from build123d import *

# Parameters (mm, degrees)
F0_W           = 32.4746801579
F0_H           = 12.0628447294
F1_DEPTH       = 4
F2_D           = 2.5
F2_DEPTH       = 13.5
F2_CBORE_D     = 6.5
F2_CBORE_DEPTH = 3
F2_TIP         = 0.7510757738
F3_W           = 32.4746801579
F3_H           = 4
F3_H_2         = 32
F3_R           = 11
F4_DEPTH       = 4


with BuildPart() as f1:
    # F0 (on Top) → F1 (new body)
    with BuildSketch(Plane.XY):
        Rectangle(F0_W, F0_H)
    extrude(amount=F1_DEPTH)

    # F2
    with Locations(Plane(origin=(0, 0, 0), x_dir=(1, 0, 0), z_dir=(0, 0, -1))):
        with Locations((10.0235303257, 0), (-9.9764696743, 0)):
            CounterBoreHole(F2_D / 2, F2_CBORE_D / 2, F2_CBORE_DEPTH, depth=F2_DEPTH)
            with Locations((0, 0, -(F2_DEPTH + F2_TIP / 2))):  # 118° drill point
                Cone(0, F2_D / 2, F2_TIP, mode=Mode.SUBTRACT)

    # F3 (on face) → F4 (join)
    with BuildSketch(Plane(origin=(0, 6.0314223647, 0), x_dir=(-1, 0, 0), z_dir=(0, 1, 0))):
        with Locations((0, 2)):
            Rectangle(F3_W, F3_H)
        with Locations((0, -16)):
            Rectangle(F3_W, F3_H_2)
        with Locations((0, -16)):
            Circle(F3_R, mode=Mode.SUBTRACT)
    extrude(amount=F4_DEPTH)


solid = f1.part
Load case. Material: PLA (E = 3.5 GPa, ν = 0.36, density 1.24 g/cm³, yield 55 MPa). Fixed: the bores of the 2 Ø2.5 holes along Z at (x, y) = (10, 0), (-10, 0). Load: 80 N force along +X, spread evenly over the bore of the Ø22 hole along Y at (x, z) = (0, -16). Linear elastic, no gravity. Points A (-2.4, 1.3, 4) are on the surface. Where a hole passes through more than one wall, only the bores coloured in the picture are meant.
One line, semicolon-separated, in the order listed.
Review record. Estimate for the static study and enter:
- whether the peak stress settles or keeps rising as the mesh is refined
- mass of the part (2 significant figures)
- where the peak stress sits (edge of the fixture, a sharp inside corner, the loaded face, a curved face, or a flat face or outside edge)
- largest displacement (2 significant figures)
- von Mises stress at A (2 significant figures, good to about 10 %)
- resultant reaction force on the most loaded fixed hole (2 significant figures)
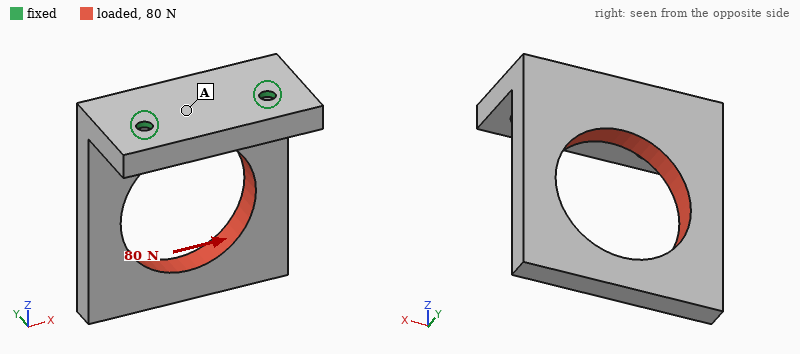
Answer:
keeps rising; 5.6 g; edge of the fixture; 0.46 mm; 4.7 MPa; 91 N
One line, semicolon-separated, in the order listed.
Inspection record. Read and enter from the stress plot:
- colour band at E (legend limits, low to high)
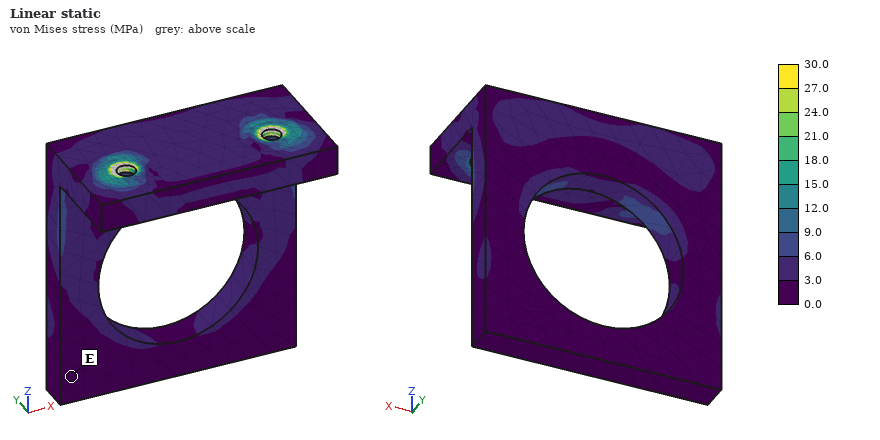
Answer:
0.0 to 3.0 MPa
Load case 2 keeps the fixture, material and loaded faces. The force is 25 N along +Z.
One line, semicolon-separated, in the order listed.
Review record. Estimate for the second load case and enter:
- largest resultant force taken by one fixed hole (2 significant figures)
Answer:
13 N
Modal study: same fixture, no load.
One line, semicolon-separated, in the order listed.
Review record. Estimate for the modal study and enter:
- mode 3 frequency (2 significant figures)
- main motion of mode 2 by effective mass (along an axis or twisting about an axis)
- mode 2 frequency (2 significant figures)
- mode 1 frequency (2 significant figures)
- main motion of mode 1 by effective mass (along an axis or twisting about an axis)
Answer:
1700 Hz; along X; 1200 Hz; 380 Hz; along Y
